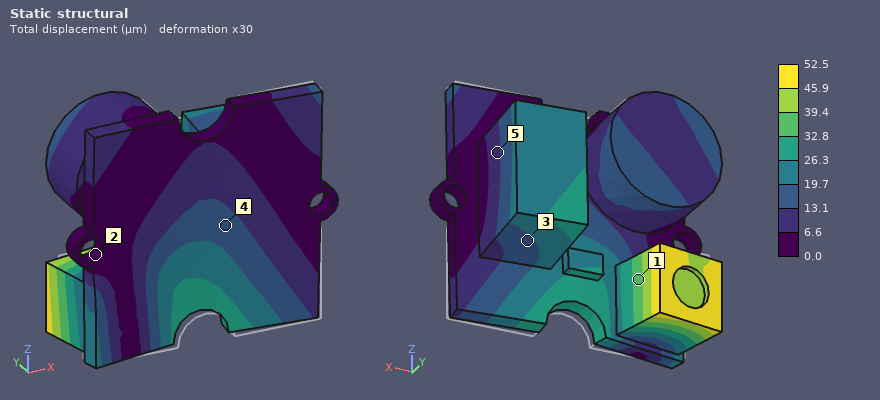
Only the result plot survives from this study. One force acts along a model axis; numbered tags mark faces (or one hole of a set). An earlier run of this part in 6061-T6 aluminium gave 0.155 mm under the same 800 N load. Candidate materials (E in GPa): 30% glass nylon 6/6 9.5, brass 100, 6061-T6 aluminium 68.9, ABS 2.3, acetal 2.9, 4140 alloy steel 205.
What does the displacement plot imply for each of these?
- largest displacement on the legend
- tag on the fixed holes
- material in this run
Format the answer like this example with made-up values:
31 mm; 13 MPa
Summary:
52.5 µm; 2; 4140 alloy steel
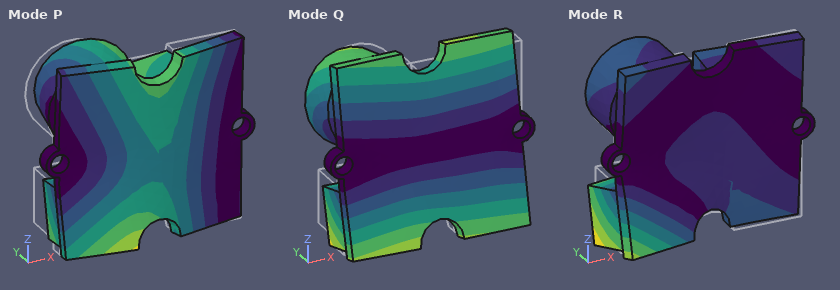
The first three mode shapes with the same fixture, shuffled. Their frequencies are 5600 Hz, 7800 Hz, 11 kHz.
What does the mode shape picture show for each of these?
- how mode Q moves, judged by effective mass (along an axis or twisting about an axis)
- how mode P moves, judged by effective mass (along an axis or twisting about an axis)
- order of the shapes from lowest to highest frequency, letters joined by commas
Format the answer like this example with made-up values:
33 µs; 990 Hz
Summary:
along Z; along Y; Q, P, R
